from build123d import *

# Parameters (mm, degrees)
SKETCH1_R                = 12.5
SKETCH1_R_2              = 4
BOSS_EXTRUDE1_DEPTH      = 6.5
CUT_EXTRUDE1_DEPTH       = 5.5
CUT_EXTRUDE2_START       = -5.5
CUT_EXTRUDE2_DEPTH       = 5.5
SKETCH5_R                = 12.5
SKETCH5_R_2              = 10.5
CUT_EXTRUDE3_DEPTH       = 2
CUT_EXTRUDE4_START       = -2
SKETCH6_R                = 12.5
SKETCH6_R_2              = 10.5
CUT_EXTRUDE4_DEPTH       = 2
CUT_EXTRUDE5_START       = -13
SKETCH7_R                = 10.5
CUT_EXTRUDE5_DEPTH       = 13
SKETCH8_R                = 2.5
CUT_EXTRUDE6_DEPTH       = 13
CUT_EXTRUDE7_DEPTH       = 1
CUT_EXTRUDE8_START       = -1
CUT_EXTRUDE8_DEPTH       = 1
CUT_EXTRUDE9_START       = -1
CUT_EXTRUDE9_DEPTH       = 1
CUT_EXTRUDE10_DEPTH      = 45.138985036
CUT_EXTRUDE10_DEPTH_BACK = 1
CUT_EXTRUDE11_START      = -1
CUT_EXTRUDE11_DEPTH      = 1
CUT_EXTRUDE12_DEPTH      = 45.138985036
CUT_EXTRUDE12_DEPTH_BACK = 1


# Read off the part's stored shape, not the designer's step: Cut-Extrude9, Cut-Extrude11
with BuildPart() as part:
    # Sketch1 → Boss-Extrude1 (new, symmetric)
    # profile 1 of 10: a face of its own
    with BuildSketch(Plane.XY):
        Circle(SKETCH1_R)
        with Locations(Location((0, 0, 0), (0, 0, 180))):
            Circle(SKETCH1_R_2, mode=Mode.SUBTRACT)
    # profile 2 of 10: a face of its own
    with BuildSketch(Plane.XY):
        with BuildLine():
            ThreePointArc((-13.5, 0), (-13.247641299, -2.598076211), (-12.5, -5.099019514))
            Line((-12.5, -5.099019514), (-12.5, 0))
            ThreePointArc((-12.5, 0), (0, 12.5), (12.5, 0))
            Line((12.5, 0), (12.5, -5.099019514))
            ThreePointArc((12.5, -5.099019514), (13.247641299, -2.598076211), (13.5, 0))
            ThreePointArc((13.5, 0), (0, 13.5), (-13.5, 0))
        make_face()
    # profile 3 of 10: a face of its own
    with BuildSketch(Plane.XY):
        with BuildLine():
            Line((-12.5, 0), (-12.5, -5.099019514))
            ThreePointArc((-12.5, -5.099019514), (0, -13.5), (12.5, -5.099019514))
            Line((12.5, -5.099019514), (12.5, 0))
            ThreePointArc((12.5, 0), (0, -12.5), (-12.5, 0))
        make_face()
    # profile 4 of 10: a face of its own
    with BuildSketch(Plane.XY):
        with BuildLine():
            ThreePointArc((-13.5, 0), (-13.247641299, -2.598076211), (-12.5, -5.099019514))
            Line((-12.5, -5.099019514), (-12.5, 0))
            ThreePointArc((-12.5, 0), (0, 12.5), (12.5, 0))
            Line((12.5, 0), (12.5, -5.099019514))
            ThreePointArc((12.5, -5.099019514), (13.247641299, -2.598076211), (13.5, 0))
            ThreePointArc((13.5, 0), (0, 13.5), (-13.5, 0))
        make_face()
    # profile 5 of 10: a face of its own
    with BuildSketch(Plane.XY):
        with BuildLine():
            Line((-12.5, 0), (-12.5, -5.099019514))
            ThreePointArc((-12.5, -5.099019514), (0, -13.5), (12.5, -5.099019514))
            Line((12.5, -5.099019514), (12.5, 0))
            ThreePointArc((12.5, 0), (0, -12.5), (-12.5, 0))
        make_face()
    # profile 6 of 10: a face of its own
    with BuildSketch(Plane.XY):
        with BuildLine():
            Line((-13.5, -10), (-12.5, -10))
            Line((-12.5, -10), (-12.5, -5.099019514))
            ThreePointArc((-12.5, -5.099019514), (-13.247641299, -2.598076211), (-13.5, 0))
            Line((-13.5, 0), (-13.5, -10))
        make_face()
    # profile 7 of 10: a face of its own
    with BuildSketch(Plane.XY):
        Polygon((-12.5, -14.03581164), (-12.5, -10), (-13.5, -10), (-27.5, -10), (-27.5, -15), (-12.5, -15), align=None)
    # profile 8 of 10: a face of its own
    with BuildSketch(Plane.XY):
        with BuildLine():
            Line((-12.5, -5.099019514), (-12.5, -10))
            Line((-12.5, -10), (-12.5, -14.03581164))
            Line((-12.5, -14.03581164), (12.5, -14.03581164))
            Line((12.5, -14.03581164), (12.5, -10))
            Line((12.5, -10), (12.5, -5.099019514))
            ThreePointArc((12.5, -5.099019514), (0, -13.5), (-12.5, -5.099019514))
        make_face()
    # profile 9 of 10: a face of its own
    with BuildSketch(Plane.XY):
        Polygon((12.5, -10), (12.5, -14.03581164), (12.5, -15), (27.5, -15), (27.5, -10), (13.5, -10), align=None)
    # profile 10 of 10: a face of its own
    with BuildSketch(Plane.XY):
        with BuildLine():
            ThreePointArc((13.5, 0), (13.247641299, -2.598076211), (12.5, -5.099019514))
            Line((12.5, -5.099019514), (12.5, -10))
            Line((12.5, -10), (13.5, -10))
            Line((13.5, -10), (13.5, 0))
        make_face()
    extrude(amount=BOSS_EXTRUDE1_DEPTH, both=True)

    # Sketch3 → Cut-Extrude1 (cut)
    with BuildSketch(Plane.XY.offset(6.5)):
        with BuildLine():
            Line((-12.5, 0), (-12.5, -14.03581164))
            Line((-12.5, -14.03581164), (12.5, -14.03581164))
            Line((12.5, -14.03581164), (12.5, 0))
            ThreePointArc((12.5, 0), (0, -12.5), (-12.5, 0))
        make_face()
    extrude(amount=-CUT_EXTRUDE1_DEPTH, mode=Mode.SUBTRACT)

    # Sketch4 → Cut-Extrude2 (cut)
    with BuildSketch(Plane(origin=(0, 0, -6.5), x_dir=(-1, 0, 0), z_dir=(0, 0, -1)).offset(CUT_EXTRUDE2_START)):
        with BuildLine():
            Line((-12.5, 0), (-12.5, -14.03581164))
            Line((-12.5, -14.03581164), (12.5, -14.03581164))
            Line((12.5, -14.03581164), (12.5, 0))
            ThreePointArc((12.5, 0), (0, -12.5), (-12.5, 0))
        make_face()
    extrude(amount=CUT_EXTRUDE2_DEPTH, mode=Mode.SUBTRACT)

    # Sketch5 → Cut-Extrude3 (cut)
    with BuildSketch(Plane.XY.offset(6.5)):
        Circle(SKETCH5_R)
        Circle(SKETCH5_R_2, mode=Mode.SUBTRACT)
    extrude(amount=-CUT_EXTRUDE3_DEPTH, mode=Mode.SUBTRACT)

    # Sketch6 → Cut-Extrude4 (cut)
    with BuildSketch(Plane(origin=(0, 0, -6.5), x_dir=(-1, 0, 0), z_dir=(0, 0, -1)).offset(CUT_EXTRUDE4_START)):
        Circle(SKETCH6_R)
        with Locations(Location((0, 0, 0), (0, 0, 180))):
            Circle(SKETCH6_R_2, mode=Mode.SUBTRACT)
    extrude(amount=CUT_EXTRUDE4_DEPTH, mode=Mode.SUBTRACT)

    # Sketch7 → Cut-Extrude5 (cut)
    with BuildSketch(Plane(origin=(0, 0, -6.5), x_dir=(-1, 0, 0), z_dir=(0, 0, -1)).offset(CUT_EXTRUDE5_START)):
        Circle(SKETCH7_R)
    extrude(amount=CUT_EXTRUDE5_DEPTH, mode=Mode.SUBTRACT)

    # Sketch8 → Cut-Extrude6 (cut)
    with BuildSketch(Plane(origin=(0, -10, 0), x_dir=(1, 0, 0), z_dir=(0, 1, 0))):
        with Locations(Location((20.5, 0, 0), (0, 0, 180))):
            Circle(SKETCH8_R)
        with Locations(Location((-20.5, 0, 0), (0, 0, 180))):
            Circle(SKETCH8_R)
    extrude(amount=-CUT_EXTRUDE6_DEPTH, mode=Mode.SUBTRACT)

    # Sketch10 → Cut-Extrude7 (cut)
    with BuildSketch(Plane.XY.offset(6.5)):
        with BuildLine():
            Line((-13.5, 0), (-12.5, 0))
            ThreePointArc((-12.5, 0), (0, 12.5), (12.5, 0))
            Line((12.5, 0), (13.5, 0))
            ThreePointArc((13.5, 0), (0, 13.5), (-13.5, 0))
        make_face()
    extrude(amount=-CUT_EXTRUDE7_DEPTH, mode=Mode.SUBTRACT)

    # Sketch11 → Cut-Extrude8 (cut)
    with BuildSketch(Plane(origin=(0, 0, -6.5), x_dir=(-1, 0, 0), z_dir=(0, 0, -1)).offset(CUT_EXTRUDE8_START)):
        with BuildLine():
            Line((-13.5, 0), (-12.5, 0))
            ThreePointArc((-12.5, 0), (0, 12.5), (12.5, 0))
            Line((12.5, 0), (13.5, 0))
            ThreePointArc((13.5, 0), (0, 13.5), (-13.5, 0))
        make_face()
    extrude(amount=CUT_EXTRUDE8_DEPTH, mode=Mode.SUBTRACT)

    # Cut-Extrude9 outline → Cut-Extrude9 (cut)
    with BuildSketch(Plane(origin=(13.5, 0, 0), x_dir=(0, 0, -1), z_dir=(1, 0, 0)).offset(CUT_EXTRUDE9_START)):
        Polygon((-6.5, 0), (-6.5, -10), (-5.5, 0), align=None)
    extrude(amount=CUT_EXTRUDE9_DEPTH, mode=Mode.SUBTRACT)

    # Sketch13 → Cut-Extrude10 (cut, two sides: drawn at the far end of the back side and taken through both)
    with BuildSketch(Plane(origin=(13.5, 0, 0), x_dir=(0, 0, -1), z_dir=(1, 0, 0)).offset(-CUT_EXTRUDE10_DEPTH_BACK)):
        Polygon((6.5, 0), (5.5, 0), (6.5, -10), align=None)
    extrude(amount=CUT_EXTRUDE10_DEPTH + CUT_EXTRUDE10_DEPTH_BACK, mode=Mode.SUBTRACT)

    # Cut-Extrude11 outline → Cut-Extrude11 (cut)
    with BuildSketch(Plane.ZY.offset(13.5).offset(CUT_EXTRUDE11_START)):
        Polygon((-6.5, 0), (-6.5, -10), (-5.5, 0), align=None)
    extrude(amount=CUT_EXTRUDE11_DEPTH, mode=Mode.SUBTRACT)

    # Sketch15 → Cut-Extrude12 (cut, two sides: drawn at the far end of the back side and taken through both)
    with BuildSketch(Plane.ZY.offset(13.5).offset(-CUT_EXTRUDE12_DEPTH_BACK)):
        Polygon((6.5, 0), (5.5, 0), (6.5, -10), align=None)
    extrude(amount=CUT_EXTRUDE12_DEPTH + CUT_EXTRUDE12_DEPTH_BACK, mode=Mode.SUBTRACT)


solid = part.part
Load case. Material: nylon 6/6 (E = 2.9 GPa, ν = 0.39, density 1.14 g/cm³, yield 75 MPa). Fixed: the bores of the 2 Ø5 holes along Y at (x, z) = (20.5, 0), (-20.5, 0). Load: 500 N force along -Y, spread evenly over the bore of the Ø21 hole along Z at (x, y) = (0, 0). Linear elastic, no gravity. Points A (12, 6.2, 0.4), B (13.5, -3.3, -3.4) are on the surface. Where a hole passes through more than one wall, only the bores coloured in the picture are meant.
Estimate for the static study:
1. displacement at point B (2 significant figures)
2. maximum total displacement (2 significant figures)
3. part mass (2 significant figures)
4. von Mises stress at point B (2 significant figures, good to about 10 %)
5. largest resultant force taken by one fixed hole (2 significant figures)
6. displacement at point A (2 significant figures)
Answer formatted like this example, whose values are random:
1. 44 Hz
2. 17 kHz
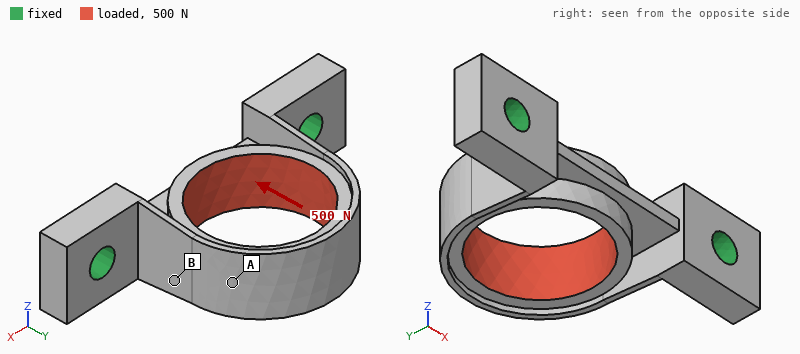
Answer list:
1. 0.13 mm
2. 0.25 mm
3. 4.5 g
4. 17 MPa
5. 260 N
6. 0.13 mm
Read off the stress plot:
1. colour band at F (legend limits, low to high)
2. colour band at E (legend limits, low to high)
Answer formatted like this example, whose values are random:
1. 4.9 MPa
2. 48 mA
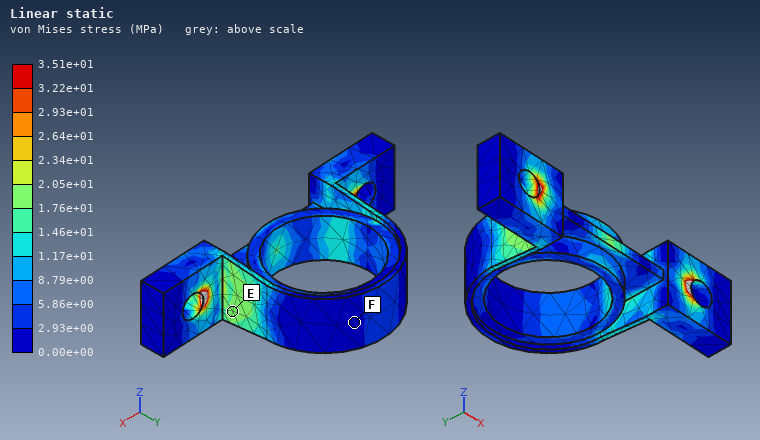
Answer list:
1. 0.00e+00 to 2.93e+00 MPa
2. 1.76e+01 to 2.05e+01 MPa
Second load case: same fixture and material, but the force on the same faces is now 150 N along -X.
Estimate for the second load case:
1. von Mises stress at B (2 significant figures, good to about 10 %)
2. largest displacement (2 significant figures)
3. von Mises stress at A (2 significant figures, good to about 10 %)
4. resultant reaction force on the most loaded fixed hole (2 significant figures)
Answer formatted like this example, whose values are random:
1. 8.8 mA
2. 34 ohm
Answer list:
1. 7.1 MPa
2. 0.32 mm
3. 6.7 MPa
4. 94 N
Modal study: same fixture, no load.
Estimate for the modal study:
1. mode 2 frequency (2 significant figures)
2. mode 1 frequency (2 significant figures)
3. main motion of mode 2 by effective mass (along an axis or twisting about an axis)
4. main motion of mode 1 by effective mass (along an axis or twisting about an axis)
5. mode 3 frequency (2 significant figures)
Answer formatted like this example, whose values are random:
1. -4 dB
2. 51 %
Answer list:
1. 2400 Hz
2. 1700 Hz
3. along X
4. along Z
5. 3700 Hz
